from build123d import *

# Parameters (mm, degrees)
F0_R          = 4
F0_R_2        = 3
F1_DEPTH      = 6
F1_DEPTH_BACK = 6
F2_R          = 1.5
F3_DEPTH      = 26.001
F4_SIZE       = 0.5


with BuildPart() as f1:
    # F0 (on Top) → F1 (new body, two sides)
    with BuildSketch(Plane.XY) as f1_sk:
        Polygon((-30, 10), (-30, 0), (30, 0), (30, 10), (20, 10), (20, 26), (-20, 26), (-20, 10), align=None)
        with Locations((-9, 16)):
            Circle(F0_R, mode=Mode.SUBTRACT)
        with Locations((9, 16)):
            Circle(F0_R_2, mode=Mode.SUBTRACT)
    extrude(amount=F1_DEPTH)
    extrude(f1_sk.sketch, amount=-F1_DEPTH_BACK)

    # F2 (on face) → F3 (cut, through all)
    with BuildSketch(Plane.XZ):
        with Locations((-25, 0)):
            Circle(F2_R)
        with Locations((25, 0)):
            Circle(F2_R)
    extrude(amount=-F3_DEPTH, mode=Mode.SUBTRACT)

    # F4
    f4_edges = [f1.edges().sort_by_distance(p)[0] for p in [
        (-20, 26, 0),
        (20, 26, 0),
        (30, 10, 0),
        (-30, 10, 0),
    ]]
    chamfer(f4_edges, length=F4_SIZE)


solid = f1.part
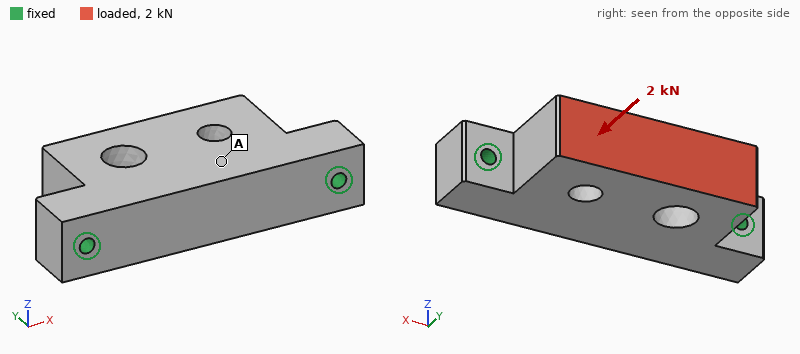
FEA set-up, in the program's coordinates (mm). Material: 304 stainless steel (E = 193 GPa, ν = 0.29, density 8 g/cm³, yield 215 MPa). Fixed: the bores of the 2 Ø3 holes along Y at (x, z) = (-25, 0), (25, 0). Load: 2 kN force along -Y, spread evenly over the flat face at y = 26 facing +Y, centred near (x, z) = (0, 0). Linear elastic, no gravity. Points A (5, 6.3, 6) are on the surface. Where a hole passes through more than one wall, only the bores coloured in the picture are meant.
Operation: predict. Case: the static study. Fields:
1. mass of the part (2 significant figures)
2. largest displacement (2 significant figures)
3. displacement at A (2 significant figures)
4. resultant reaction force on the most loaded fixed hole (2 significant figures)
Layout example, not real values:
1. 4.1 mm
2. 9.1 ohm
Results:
1. 110 g
2. 2.8 µm
3. 2.4 µm
4. 1.1 kN
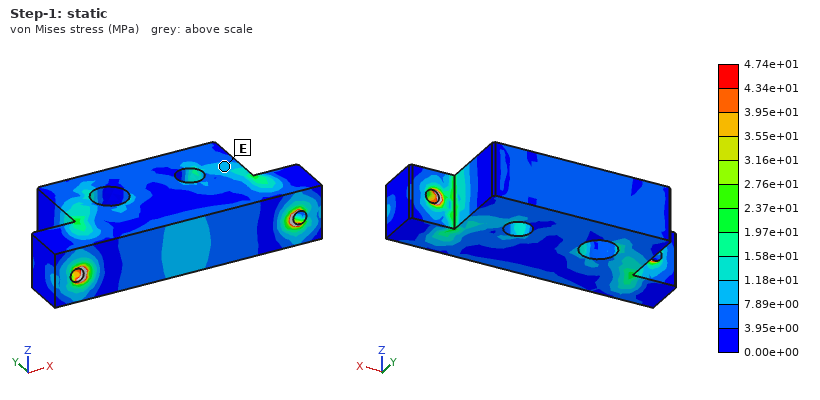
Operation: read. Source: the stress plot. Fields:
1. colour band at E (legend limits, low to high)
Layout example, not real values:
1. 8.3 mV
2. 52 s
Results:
1. 7.89e+00 to 1.18e+01 MPa
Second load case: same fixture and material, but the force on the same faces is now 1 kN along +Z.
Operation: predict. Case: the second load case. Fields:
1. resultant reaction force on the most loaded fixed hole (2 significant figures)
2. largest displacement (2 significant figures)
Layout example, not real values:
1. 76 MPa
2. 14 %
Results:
1. 500 N
2. 19 µm
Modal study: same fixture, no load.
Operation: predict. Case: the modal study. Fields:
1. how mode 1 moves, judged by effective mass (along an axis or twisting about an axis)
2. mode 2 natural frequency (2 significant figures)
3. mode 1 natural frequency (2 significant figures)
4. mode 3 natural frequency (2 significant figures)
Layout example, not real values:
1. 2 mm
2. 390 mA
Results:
1. along Z
2. 16 kHz
3. 7000 Hz
4. 16 kHz
